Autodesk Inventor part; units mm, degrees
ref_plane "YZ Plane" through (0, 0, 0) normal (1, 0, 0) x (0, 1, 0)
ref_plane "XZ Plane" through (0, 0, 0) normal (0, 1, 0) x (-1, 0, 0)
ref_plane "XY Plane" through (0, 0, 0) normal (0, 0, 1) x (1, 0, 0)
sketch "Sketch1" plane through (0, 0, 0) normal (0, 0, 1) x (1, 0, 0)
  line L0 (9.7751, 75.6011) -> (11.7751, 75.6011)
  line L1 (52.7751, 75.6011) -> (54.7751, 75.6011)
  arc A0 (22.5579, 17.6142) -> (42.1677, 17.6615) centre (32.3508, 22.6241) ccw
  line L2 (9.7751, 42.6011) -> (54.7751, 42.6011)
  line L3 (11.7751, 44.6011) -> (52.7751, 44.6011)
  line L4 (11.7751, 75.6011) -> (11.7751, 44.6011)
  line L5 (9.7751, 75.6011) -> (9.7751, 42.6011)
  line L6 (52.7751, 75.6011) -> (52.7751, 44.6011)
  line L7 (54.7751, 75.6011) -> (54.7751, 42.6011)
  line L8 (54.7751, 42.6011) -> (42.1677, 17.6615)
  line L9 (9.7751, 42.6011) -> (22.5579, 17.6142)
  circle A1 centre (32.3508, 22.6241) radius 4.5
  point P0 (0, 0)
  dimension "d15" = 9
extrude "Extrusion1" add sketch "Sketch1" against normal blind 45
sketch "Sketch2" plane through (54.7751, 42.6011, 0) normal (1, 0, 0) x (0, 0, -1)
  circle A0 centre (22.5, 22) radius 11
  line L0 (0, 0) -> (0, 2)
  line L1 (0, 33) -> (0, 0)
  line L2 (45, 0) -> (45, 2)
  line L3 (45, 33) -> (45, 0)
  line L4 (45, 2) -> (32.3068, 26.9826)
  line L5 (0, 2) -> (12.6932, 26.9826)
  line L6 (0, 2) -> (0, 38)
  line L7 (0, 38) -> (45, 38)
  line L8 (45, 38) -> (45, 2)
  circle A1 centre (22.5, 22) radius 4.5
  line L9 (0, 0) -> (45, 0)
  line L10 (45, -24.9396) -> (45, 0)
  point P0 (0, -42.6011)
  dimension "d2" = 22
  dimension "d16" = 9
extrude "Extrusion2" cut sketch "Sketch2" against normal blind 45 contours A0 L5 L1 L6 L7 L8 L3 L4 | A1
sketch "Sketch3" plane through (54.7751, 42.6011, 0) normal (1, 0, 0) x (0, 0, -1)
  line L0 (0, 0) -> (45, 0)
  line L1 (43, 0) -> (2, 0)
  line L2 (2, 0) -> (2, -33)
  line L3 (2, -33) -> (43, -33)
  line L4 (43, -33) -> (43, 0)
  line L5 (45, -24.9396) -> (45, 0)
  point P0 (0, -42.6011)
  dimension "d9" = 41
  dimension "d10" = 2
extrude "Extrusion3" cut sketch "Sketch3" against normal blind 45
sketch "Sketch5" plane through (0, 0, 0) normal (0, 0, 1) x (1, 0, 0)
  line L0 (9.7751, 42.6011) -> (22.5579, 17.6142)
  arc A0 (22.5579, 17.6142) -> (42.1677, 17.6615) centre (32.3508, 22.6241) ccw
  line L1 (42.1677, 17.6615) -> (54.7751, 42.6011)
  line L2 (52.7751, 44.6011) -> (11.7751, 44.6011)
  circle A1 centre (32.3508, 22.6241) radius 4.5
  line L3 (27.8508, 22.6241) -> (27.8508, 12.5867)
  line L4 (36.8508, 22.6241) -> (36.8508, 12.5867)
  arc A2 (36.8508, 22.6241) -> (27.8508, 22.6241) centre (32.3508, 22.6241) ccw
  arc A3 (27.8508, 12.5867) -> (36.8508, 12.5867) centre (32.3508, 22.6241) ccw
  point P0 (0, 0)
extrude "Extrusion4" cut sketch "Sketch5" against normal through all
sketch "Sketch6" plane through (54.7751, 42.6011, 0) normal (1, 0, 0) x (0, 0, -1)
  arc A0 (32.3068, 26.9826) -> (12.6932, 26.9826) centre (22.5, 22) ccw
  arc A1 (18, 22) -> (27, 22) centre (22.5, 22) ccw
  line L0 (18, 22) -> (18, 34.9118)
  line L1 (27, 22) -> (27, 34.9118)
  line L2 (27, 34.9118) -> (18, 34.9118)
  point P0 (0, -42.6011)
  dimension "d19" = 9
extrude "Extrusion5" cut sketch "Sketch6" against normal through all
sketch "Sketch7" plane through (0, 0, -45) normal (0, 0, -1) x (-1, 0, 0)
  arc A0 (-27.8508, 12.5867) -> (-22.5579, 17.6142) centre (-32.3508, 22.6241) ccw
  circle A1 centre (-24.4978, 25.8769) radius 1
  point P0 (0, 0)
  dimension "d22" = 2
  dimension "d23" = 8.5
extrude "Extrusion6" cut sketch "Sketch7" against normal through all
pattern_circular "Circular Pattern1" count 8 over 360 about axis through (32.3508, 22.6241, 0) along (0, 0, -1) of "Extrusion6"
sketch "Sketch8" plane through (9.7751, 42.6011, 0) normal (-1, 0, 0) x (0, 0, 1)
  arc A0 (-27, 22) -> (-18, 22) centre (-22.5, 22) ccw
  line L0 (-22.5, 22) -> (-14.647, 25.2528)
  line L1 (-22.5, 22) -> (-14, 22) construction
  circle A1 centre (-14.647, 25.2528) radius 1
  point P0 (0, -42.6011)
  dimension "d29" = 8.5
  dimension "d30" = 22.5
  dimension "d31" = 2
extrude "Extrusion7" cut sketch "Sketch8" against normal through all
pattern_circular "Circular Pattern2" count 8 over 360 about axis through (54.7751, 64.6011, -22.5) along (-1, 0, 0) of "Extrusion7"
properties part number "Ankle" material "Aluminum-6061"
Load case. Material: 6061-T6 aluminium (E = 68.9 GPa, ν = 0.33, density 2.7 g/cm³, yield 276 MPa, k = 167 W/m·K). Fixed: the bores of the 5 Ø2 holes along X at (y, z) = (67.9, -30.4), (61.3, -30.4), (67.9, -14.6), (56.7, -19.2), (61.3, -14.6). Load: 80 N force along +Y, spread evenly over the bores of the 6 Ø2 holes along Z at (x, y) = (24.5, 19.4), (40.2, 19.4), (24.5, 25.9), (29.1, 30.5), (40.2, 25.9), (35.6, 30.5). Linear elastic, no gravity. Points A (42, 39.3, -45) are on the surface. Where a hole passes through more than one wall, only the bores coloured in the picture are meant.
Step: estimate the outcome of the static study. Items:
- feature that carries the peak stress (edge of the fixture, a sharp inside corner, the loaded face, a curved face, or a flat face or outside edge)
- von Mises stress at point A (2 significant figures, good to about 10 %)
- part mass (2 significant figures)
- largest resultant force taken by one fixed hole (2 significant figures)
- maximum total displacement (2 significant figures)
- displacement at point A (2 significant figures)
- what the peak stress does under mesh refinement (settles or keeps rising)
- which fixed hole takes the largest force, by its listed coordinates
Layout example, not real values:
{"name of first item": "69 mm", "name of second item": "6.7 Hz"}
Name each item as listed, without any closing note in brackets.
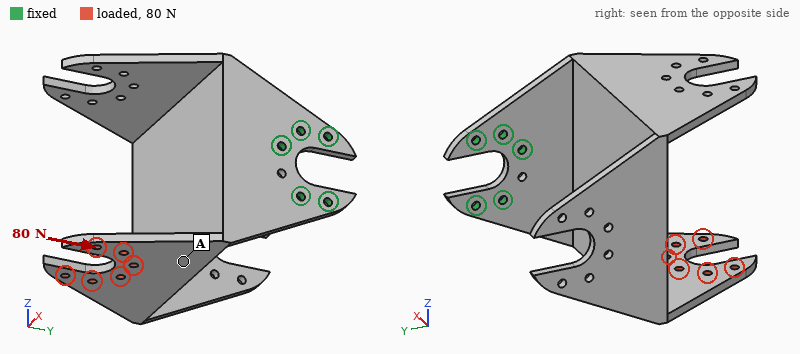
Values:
{"feature that carries the peak stress": "edge of the fixture", "von Mises stress at point A": "13 MPa", "part mass": "27 g", "largest resultant force taken by one fixed hole": "150 N", "maximum total displacement": "0.98 mm", "displacement at point A": "0.35 mm", "what the peak stress does under mesh refinement": "keeps rising", "which fixed hole takes the largest force, by its listed coordinates": "(56.7, -19.2)"}
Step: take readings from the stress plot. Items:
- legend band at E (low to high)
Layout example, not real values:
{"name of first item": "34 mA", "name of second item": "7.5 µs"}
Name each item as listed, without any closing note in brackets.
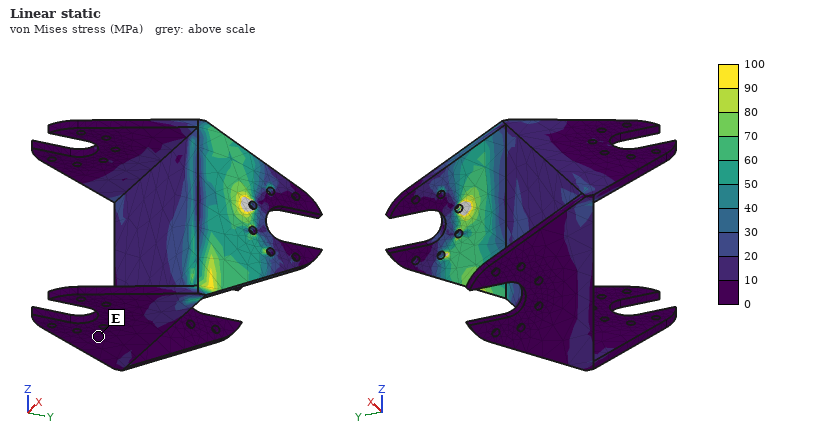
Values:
{"legend band at E": "0 to 10 MPa"}
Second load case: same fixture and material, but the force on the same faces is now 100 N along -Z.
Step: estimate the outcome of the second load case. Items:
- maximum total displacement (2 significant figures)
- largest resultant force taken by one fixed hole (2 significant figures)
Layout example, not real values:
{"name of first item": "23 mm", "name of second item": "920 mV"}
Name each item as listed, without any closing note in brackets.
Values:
{"maximum total displacement": "0.62 mm", "largest resultant force taken by one fixed hole": "170 N"}
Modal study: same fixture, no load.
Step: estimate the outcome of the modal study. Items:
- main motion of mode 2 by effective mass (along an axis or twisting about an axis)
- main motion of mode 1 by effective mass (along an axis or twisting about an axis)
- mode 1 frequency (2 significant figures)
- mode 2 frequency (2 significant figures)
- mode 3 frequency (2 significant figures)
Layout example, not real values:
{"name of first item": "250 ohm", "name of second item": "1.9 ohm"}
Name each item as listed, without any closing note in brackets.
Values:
{"main motion of mode 2 by effective mass": "along Z", "main motion of mode 1 by effective mass": "along Y", "mode 1 frequency": "330 Hz", "mode 2 frequency": "550 Hz", "mode 3 frequency": "1000 Hz"}
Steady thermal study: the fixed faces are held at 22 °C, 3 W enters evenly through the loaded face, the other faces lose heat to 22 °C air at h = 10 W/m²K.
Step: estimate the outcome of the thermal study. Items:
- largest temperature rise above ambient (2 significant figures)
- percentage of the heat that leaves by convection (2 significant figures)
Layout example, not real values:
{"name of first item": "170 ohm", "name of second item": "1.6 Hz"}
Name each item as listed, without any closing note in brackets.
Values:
{"largest temperature rise above ambient": "14 K", "percentage of the heat that leaves by convection": "20 %"}
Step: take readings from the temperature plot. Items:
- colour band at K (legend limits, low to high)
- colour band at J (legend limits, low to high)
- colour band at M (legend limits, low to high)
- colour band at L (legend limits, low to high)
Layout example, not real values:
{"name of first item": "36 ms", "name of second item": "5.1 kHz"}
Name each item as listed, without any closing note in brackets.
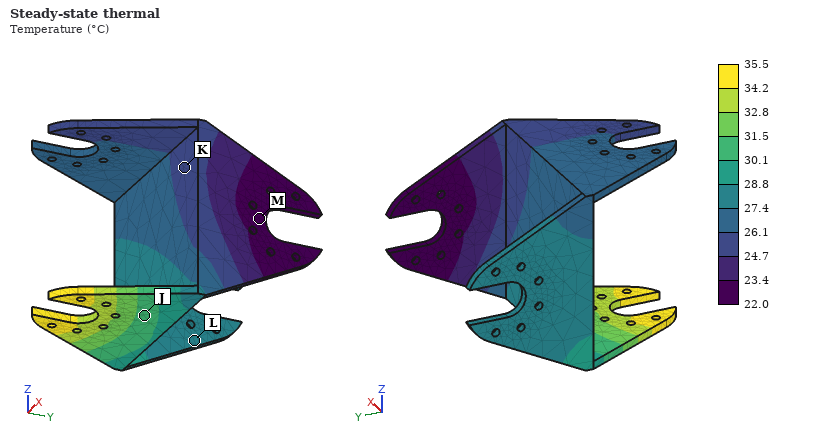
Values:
{"colour band at K": "24.7 to 26.1 °C", "colour band at J": "30.1 to 31.5 °C", "colour band at M": "22.0 to 23.4 °C", "colour band at L": "27.4 to 28.8 °C"}
